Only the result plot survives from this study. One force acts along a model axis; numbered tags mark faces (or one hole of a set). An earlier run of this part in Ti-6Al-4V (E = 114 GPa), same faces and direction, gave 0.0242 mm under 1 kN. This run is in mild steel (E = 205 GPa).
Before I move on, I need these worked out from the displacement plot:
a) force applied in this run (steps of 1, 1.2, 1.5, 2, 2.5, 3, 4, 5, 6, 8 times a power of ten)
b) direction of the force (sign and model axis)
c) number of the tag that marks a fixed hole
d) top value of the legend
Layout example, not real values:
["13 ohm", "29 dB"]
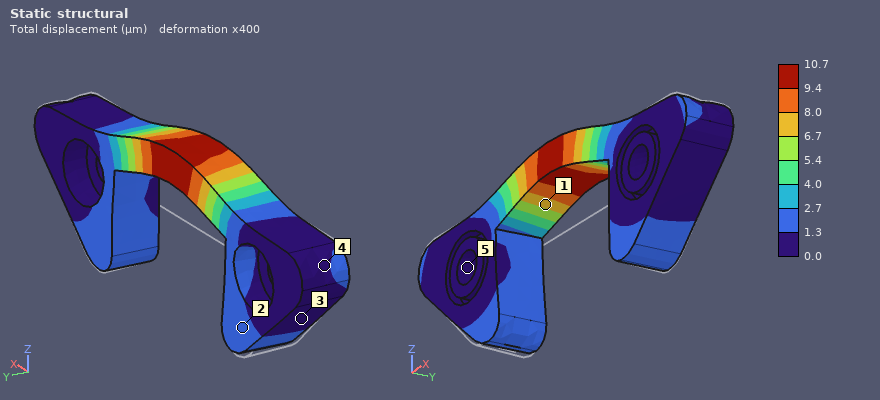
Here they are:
["800 N", "+Z", "5", "10.7 µm"]
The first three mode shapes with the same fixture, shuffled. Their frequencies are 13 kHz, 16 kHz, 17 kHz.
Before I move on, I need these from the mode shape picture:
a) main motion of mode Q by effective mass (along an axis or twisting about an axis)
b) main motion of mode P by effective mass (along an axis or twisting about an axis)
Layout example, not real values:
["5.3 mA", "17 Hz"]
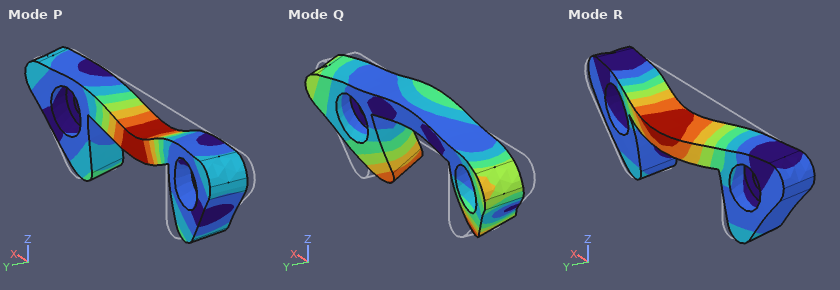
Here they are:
["twisting about X", "along Z"]
